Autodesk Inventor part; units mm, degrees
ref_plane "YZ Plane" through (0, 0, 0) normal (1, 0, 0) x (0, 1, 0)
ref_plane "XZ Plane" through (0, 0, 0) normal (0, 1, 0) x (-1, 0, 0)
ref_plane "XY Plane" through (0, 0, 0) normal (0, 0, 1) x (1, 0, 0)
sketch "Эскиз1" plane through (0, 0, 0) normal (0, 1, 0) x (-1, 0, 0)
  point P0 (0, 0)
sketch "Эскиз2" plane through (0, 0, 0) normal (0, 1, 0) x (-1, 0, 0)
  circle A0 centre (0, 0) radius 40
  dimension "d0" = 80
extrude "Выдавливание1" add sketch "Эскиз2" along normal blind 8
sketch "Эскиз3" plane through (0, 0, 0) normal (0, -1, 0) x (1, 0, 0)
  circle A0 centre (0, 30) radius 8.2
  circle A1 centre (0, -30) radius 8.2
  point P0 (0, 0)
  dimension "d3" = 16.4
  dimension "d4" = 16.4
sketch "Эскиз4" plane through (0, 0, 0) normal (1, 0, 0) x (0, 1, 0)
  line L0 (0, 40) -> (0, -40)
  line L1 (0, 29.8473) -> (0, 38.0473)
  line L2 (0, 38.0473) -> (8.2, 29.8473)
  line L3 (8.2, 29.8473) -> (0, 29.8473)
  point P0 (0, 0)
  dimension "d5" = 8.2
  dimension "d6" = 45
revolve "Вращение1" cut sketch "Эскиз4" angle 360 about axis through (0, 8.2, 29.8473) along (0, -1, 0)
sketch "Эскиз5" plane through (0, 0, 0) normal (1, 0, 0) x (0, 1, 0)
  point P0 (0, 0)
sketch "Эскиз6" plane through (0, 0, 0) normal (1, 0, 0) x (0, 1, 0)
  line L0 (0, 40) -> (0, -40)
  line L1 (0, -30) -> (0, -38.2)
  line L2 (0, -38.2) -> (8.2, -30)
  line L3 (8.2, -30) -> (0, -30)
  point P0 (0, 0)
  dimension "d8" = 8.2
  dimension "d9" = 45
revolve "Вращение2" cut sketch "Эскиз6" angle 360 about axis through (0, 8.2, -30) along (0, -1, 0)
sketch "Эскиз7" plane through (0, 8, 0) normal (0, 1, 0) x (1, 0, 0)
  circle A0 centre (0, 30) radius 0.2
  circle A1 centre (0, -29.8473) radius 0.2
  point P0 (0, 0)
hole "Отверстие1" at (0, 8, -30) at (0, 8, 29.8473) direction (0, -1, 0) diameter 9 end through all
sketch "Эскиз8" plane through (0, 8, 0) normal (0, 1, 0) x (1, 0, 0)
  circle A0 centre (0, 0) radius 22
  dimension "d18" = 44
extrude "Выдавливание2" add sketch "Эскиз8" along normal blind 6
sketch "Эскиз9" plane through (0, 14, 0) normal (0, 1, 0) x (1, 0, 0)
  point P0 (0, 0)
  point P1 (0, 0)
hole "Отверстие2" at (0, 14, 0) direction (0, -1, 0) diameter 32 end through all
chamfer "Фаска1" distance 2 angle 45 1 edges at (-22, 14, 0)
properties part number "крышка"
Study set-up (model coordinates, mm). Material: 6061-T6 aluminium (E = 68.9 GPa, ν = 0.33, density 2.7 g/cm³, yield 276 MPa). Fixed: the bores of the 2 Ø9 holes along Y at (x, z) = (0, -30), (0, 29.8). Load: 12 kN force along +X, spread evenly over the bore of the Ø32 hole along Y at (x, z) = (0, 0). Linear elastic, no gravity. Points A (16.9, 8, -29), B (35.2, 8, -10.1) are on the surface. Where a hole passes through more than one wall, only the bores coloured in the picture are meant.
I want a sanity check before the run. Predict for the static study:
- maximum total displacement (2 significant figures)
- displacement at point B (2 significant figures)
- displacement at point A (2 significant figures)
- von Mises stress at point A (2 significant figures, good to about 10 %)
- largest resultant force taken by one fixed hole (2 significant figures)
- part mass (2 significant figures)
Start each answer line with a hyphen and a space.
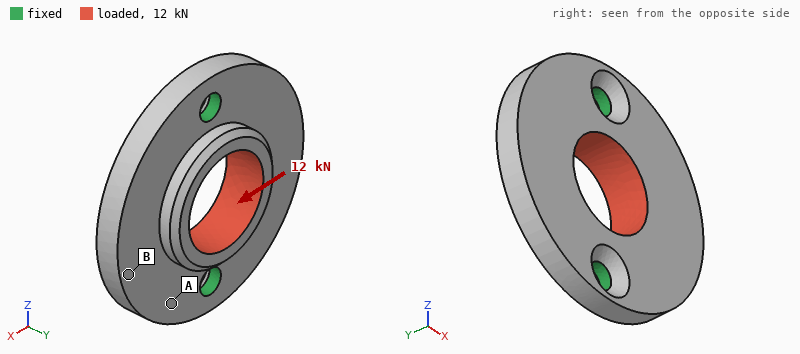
- 52 µm
- 44 µm
- 13 µm
- 23 MPa
- 6.0 kN
- 98 g
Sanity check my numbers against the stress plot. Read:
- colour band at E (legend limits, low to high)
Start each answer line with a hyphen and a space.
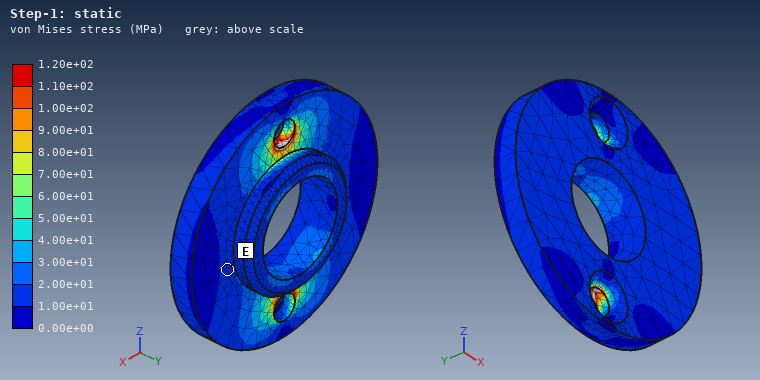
- 1.00e+01 to 2.00e+01 MPa
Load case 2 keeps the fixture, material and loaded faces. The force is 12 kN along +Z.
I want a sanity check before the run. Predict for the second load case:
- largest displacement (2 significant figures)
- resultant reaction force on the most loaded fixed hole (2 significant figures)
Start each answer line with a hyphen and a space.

- 17 µm
- 6.0 kN
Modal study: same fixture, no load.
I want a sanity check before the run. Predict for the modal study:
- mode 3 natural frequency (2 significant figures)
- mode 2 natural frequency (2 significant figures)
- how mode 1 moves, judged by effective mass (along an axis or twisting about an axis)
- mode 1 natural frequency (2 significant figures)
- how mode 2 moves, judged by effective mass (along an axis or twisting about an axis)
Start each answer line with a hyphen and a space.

- 9100 Hz
- 4500 Hz
- twisting about Z
- 3200 Hz
- along Y
